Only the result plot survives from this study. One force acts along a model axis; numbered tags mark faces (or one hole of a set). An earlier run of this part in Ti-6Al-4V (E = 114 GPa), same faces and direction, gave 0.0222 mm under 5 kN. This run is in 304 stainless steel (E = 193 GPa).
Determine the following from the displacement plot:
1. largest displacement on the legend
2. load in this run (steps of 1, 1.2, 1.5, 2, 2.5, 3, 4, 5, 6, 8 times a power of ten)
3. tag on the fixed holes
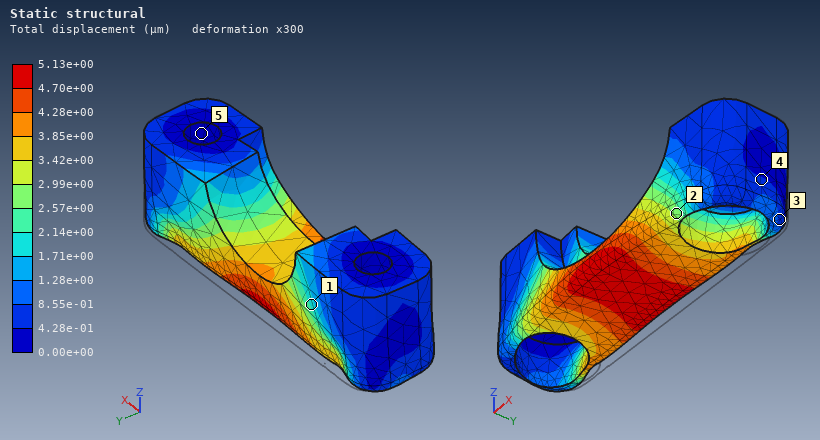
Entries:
5.13e+00 µm
2 kN
5
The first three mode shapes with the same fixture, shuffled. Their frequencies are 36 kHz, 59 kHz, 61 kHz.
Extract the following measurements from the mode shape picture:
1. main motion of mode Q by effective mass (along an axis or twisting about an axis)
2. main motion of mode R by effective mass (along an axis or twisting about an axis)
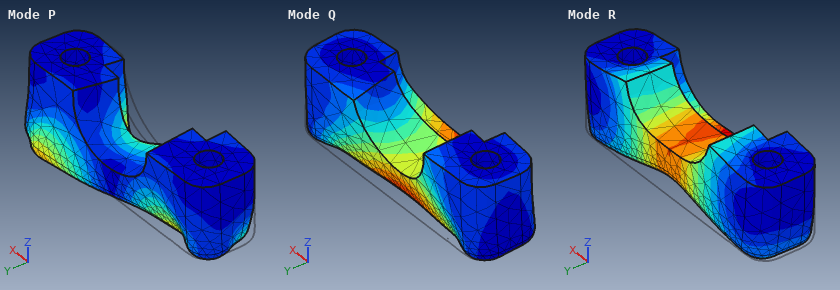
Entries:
along Y
along Z
